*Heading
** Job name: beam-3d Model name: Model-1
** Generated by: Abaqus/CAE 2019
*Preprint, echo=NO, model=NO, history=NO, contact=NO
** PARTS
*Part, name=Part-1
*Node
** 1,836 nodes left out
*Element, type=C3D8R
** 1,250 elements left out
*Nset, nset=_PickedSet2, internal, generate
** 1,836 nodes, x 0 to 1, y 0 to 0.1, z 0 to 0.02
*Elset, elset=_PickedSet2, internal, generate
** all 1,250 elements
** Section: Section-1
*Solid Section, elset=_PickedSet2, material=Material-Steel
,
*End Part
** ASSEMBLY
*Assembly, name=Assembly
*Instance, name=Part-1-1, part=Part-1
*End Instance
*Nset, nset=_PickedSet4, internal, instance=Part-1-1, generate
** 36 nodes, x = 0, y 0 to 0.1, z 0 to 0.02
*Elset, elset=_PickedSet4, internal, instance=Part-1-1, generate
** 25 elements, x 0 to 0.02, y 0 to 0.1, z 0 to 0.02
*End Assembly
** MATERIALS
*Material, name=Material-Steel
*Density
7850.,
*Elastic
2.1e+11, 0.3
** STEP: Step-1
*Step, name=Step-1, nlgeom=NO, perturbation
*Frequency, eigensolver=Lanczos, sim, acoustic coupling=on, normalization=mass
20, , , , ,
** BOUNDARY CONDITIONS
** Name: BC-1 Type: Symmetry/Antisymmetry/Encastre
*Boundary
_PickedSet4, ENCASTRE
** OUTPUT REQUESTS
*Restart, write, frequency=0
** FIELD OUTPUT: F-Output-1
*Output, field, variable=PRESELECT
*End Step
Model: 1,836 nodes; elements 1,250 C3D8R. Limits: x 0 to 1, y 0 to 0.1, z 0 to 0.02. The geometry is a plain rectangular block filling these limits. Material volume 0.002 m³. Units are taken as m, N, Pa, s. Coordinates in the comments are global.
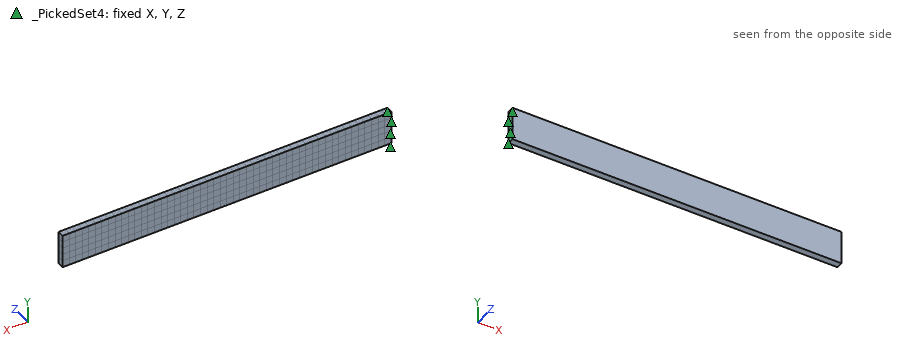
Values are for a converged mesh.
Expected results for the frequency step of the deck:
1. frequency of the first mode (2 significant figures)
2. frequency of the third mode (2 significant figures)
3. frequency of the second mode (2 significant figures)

17 Hz
110 Hz
83 Hz
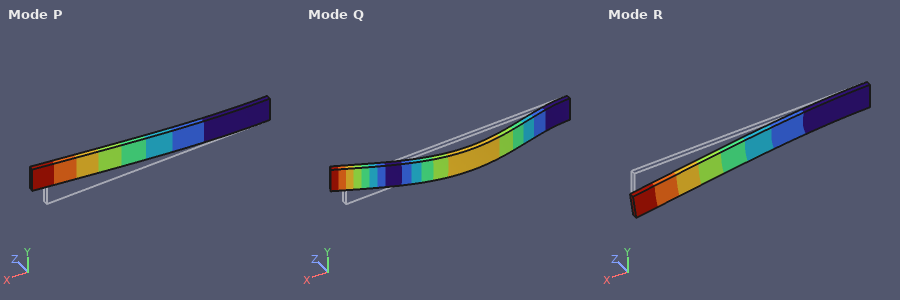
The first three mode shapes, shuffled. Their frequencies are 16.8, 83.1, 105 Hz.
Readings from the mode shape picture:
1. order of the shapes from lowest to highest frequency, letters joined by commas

P, R, Q
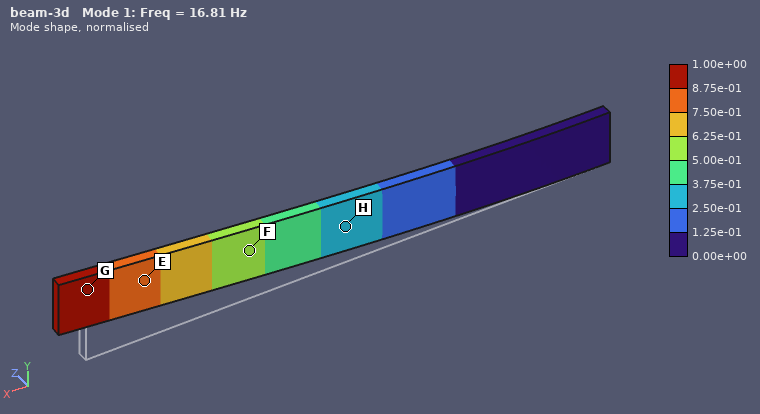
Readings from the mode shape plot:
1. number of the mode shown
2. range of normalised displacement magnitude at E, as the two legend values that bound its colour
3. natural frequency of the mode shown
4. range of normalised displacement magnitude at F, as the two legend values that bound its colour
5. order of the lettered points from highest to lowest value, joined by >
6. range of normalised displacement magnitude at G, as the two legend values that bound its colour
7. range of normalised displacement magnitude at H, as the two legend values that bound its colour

1
7.50e-01 to 8.75e-01
16.81 Hz
5.00e-01 to 6.25e-01
G > E > F > H
8.75e-01 to 1.00e+00
2.50e-01 to 3.75e-01
